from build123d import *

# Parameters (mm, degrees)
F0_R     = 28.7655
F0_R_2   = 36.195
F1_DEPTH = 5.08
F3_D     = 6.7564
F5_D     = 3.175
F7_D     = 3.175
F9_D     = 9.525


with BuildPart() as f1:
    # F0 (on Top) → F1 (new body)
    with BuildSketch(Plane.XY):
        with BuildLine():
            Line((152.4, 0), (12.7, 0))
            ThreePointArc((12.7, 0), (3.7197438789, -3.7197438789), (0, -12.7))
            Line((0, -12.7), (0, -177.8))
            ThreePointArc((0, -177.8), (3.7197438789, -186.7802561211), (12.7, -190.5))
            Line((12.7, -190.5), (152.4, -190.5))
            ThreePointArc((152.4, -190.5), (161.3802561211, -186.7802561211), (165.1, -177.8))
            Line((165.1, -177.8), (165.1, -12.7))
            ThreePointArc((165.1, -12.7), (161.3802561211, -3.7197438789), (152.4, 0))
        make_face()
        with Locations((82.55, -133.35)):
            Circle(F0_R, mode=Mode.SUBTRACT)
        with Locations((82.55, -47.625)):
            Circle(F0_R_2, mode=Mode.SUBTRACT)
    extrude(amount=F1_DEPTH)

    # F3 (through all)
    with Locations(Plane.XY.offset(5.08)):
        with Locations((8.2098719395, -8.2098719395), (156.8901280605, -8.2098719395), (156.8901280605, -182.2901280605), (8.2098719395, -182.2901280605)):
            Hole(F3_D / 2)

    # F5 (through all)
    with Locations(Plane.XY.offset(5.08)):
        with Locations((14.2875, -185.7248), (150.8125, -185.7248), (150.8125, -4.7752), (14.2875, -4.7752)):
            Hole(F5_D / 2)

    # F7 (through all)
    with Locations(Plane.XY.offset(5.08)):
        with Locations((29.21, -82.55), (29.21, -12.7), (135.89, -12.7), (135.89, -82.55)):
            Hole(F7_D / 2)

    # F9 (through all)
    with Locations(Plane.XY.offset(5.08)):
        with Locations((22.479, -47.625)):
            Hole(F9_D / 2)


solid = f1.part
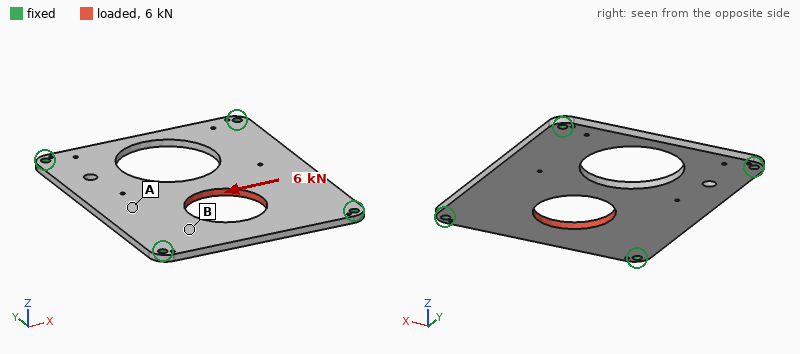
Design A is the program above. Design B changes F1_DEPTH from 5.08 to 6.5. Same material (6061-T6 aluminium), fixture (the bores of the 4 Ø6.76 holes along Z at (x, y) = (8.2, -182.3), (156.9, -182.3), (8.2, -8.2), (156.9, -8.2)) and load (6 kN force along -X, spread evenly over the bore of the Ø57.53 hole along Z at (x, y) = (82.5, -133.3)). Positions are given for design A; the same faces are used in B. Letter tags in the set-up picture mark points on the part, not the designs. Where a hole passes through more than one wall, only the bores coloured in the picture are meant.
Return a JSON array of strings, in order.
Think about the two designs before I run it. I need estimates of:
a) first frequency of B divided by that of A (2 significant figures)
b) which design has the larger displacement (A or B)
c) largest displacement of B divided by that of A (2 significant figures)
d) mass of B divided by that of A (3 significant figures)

["1.3", "A", "0.78", "1.28"]
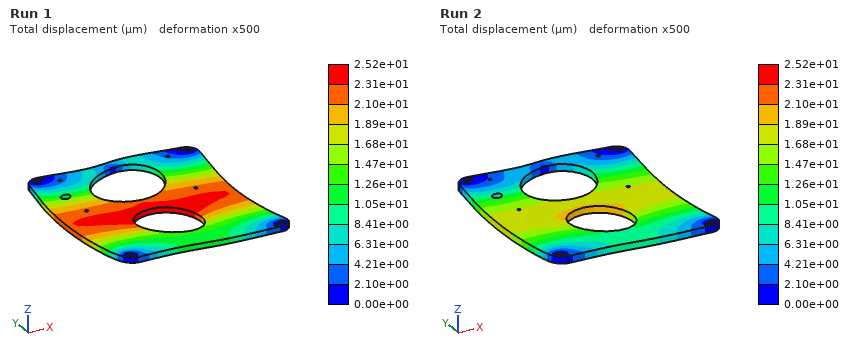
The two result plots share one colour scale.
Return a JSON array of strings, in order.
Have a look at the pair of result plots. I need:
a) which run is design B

["Run 2"]
